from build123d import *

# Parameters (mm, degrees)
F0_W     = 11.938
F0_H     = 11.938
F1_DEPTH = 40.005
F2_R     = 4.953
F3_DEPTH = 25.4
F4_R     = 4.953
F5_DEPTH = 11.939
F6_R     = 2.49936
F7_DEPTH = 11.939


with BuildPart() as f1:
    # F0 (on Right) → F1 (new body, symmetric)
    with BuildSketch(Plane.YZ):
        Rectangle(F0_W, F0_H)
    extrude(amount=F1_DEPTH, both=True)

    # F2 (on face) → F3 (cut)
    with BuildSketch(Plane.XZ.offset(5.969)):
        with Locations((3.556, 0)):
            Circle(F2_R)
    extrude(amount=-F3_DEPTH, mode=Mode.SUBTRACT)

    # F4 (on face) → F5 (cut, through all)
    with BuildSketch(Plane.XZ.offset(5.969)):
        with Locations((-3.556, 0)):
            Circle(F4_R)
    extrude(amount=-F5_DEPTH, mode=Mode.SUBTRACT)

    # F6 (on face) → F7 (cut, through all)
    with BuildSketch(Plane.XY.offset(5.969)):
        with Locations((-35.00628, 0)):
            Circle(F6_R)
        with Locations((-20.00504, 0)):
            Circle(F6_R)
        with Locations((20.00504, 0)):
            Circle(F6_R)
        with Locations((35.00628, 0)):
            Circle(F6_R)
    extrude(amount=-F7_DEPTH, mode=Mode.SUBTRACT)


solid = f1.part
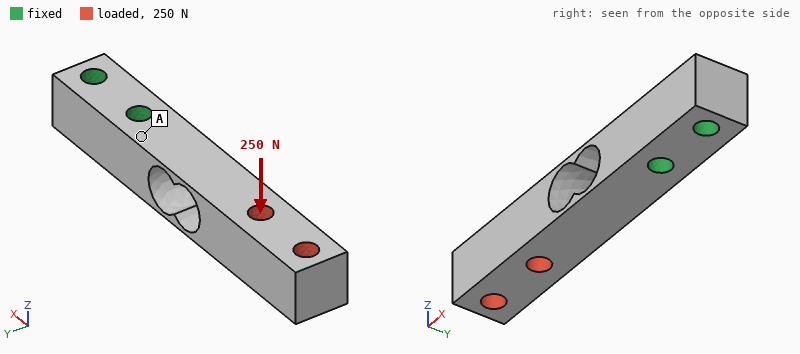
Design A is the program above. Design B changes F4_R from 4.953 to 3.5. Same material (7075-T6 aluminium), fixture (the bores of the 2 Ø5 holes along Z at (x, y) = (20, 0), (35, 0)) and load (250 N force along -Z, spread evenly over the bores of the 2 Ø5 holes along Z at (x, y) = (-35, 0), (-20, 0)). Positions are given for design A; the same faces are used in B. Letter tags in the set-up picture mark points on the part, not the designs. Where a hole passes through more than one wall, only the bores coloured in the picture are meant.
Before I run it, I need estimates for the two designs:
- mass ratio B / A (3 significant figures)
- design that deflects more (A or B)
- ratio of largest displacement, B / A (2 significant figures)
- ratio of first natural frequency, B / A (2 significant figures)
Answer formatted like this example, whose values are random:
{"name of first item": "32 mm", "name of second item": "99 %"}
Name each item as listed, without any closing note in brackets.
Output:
{"mass ratio B / A": "1.04", "design that deflects more": "A", "ratio of largest displacement, B / A": "0.49", "ratio of first natural frequency, B / A": "1.3"}
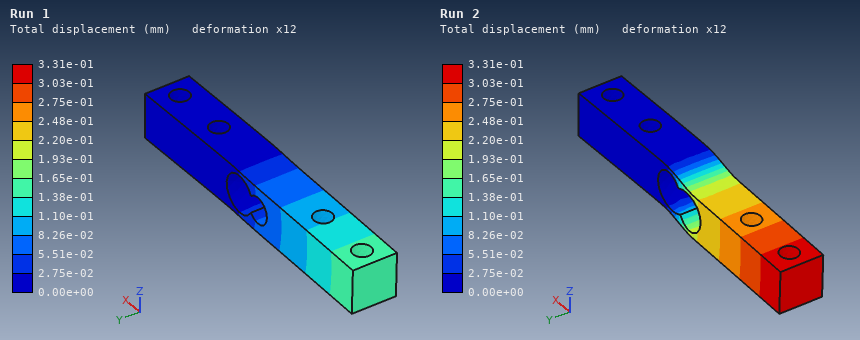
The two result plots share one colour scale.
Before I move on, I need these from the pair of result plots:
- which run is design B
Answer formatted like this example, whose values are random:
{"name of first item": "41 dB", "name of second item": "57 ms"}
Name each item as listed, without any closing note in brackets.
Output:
{"which run is design B": "Run 1"}
